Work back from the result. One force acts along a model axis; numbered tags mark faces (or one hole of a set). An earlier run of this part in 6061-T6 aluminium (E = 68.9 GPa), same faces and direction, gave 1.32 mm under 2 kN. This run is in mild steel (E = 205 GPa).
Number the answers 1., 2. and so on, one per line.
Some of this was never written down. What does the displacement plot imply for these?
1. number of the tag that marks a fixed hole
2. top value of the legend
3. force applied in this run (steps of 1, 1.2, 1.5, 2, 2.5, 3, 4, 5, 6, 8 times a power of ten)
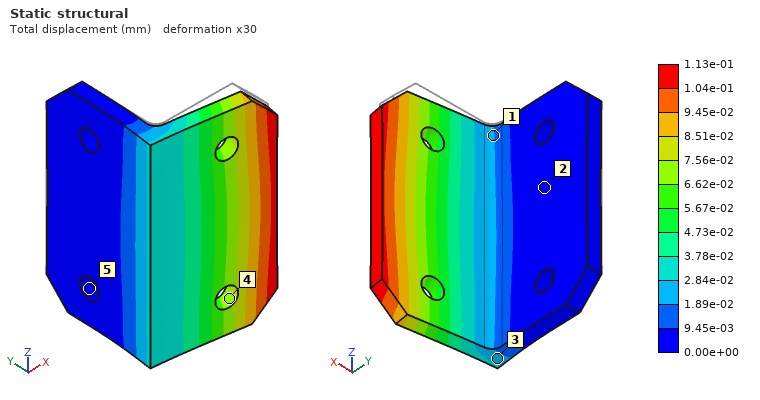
1. 5
2. 1.13e-01 mm
3. 500 N
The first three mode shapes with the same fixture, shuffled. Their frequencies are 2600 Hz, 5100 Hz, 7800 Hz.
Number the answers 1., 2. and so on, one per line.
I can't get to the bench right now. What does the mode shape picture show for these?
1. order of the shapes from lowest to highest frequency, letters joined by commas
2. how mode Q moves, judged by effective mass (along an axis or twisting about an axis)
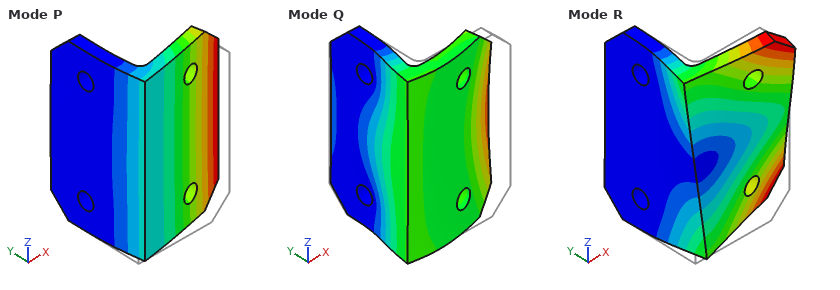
1. P, R, Q
2. along X
